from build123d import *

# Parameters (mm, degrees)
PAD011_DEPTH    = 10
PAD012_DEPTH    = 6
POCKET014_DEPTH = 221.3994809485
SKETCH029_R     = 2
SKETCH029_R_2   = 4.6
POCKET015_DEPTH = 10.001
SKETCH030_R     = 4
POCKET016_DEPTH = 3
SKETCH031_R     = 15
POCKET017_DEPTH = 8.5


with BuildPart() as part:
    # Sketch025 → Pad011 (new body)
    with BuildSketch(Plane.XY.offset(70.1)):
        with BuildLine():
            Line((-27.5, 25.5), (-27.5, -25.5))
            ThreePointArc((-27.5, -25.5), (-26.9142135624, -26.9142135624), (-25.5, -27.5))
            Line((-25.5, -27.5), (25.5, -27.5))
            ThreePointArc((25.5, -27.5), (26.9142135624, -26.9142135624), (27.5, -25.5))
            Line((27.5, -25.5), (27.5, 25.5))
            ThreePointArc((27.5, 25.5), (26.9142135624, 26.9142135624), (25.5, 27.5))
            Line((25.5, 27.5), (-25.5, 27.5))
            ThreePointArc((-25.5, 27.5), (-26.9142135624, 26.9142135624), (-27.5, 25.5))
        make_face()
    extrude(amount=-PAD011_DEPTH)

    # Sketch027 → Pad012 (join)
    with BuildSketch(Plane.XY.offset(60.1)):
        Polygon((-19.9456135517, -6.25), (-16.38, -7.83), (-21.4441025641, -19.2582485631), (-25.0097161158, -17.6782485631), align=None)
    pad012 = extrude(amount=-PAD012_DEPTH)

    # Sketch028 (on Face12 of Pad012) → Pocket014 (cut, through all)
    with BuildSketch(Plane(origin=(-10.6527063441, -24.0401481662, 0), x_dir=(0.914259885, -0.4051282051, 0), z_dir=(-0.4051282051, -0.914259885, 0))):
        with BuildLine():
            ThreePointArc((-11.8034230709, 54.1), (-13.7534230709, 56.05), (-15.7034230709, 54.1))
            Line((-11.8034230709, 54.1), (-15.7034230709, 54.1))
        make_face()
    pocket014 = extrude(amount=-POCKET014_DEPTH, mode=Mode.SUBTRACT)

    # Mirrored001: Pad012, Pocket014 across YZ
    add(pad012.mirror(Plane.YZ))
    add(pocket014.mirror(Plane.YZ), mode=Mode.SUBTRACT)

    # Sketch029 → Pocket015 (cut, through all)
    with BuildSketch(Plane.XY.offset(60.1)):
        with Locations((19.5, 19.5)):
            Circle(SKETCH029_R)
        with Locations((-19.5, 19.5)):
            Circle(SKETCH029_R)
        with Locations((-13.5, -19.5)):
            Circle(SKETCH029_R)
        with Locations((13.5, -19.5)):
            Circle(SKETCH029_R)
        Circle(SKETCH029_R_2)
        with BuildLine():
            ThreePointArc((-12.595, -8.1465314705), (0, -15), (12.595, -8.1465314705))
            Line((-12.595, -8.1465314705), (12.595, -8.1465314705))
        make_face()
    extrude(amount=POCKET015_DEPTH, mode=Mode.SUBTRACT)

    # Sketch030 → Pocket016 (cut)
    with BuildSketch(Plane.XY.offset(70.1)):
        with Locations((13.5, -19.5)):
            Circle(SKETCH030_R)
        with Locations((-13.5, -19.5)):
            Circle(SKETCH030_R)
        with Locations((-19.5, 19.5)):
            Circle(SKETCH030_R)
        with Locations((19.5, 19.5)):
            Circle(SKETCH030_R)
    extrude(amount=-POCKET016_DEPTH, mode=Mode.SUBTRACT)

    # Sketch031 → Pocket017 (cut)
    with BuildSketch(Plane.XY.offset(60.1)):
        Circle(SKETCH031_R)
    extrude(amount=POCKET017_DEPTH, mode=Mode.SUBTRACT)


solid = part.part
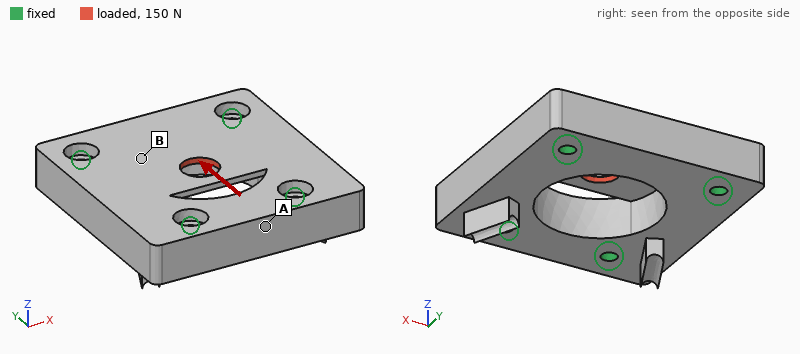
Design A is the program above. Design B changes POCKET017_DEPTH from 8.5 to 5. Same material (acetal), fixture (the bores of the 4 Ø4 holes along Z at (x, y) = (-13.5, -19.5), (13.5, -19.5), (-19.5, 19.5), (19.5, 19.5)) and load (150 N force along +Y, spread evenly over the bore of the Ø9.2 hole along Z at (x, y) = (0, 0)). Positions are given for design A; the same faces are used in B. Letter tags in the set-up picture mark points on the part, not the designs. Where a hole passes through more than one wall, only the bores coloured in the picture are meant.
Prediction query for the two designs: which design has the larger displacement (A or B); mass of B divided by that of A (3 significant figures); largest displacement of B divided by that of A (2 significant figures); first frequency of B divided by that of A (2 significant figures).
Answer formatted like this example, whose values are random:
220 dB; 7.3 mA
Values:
A; 1.08; 0.35; 1.5
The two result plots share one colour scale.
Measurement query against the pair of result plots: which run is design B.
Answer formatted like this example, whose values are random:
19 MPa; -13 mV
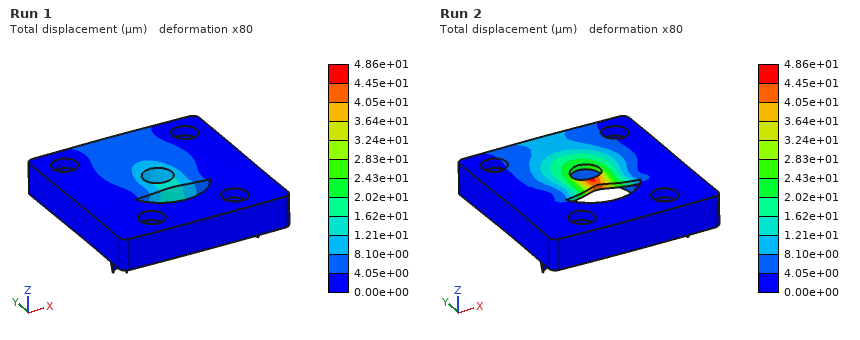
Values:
Run 1
